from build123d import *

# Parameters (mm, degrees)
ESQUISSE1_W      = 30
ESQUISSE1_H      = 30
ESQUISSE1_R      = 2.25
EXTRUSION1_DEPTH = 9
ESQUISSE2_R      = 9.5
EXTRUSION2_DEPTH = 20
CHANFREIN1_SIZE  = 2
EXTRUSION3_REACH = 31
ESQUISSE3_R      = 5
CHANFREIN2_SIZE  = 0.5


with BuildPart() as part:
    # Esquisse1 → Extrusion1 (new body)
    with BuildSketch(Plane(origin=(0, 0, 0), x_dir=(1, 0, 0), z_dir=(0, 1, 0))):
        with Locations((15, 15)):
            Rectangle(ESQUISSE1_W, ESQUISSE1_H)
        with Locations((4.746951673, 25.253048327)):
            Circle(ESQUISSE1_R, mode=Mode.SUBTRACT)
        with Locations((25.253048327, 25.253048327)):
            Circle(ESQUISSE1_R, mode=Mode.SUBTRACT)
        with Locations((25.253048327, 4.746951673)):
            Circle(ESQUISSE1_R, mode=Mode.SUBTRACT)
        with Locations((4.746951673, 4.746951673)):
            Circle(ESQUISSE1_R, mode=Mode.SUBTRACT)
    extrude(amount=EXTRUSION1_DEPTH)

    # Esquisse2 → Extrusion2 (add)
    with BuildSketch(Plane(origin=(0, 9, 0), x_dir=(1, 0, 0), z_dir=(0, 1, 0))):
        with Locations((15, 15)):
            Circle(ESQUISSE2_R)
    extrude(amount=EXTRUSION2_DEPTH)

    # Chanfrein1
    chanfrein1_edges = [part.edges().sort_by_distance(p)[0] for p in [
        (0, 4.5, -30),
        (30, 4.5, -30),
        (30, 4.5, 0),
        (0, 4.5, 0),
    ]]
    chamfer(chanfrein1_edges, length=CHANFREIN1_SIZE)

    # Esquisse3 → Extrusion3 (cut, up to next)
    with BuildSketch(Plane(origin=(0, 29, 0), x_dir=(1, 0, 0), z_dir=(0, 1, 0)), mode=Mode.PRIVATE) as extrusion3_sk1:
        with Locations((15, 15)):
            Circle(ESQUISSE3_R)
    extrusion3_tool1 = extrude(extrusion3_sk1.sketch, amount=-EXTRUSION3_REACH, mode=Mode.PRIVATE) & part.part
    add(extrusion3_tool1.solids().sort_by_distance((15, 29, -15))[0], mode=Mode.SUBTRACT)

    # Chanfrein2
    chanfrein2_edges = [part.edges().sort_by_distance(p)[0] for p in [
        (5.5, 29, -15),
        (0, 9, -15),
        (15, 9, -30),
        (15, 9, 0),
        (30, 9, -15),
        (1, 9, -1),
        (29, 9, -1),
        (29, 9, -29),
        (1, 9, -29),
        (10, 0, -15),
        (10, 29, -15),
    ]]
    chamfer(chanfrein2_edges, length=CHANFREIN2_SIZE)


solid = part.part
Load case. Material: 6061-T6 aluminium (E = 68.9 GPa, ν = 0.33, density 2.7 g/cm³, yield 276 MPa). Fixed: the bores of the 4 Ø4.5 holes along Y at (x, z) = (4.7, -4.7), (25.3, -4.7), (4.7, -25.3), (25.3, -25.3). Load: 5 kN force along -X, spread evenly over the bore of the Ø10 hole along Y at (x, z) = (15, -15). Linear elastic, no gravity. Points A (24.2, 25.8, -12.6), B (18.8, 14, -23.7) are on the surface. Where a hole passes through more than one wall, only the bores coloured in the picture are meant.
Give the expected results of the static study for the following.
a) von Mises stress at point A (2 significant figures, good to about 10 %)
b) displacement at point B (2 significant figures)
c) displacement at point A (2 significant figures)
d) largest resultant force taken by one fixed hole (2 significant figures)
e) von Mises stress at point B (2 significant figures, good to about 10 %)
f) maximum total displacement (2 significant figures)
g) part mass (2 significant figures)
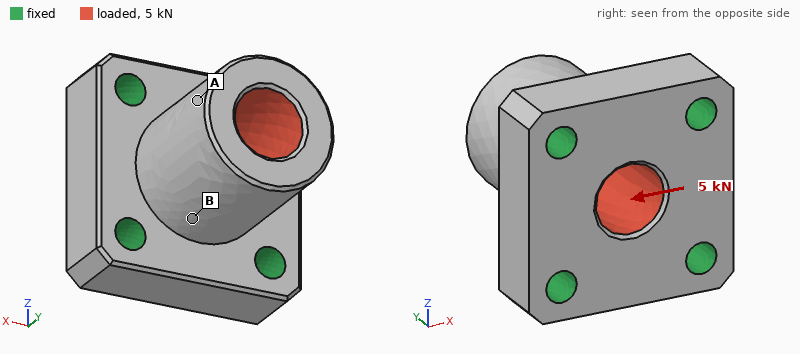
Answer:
7.8 MPa
11 µm
29 µm
1.8 kN
27 MPa
33 µm
29 g
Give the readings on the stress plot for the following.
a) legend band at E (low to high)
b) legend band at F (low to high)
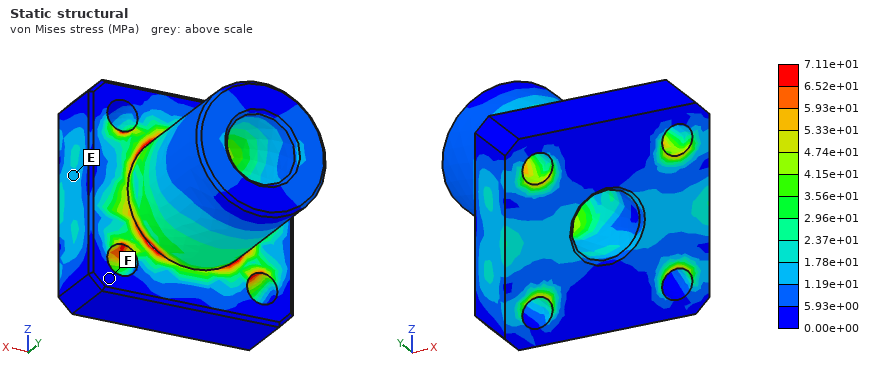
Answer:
1.19e+01 to 1.78e+01 MPa
0.00e+00 to 5.93e+00 MPa
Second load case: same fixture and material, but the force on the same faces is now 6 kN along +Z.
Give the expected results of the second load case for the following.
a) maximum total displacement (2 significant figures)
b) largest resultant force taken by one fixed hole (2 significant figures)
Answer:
39 µm
2.2 kN
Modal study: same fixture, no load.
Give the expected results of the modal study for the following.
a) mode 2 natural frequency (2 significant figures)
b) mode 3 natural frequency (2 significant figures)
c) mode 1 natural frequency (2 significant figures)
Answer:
18 kHz
34 kHz
18 kHz
